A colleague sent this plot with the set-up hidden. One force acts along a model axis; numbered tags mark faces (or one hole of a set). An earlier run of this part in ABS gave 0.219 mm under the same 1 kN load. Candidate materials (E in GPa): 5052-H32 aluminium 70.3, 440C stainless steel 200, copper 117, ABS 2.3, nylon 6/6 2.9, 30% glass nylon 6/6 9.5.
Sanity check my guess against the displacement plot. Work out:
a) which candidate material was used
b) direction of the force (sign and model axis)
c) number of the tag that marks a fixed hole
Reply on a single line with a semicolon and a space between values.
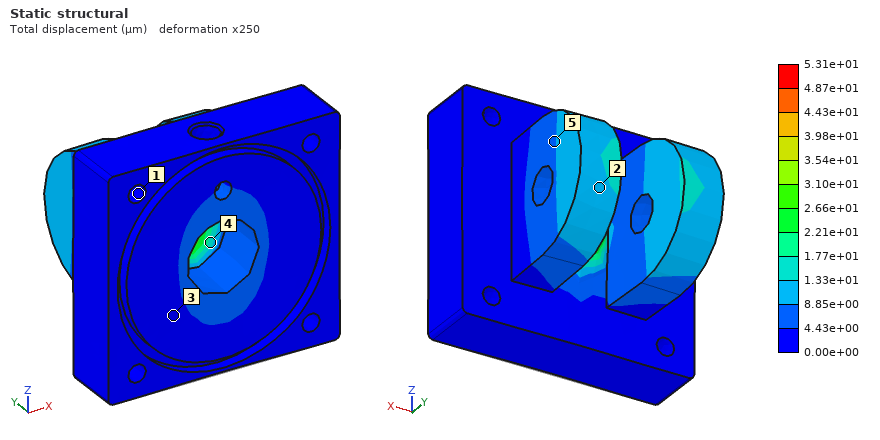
30% glass nylon 6/6; +Y; 1
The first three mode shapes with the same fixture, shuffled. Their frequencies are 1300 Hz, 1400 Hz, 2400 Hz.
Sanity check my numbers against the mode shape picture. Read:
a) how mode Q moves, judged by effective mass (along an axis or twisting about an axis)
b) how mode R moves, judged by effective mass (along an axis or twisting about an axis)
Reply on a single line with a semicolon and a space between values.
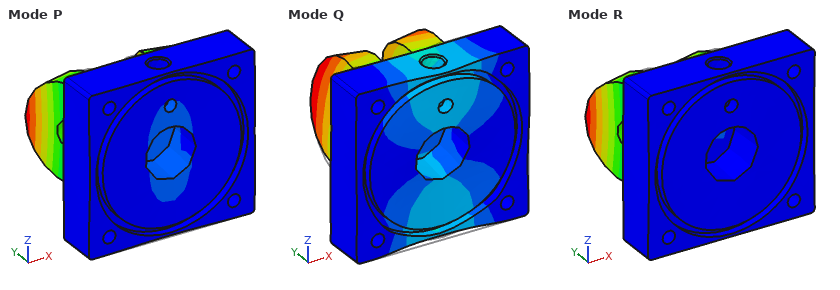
along Z; along X
